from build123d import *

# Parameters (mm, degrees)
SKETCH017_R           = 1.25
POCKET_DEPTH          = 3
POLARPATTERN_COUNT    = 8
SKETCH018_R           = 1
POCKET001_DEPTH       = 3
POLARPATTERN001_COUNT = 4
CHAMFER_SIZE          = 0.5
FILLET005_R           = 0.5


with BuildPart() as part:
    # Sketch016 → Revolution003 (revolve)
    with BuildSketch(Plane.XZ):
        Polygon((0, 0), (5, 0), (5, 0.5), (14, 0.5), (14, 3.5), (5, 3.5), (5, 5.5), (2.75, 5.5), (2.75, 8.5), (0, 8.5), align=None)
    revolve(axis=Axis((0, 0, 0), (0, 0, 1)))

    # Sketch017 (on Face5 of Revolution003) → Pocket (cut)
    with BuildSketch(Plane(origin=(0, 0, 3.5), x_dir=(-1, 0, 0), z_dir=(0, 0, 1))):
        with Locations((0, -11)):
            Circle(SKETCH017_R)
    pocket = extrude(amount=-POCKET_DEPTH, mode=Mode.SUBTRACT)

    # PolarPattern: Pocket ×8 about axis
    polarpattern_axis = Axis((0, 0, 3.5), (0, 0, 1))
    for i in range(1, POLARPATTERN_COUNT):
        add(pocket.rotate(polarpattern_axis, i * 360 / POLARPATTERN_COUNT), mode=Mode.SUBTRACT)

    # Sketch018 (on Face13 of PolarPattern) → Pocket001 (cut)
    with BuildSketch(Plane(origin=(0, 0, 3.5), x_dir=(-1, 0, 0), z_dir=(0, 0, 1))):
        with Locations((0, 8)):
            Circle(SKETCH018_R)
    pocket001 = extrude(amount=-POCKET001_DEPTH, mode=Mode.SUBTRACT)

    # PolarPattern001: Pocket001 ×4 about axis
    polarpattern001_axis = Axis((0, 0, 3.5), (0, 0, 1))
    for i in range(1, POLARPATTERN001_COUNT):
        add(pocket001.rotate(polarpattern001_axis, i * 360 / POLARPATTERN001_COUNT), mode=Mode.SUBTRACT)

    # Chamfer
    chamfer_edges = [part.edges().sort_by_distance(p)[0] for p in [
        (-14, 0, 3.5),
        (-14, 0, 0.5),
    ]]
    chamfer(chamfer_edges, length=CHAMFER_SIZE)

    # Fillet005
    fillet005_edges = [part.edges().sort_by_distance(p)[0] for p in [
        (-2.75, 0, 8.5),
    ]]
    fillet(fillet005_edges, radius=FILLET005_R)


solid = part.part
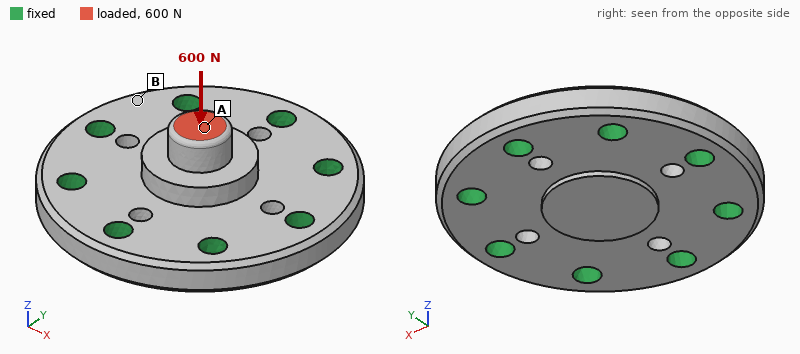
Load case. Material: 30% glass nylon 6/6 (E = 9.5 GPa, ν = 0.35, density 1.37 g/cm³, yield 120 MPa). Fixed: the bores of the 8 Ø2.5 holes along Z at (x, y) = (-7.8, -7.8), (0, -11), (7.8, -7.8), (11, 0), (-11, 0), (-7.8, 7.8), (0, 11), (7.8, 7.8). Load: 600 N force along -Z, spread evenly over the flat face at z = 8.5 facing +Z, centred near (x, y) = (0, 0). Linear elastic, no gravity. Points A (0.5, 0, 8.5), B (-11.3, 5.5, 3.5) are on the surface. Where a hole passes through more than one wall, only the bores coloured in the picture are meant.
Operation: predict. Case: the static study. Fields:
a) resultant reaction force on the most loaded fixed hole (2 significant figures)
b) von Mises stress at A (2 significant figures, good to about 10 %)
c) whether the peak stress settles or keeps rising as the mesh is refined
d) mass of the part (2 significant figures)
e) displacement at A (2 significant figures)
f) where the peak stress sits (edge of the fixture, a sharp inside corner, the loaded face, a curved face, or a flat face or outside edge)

89 N
23 MPa
keeps rising
2.7 g
41 µm
edge of the fixture
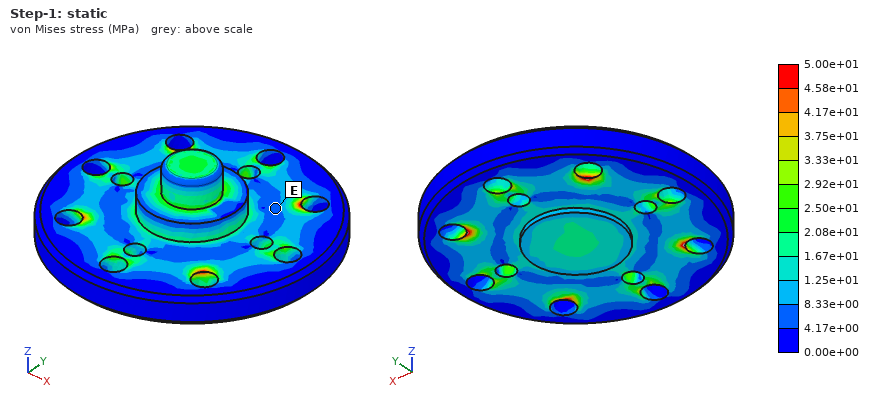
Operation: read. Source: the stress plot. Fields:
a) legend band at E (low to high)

4.17e+00 to 8.33e+00 MPa
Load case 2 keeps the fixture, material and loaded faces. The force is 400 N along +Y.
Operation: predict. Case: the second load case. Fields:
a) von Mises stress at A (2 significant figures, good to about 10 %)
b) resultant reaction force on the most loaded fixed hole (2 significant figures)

44 MPa
100 N
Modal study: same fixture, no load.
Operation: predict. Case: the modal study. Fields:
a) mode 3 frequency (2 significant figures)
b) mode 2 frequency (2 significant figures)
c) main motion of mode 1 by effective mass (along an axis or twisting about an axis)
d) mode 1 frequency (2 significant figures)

38 kHz
38 kHz
along Z
25 kHz
